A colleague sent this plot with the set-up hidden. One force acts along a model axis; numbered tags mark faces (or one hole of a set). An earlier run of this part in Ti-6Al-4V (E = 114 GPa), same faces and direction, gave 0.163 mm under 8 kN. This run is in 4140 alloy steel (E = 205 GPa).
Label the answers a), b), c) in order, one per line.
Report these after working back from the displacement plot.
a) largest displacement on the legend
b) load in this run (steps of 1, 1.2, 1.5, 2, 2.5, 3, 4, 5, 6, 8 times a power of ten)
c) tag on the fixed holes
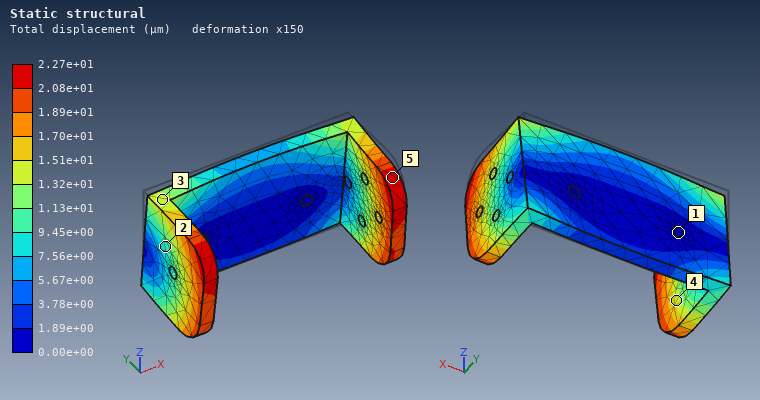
a) 2.27e+01 µm
b) 2 kN
c) 1
